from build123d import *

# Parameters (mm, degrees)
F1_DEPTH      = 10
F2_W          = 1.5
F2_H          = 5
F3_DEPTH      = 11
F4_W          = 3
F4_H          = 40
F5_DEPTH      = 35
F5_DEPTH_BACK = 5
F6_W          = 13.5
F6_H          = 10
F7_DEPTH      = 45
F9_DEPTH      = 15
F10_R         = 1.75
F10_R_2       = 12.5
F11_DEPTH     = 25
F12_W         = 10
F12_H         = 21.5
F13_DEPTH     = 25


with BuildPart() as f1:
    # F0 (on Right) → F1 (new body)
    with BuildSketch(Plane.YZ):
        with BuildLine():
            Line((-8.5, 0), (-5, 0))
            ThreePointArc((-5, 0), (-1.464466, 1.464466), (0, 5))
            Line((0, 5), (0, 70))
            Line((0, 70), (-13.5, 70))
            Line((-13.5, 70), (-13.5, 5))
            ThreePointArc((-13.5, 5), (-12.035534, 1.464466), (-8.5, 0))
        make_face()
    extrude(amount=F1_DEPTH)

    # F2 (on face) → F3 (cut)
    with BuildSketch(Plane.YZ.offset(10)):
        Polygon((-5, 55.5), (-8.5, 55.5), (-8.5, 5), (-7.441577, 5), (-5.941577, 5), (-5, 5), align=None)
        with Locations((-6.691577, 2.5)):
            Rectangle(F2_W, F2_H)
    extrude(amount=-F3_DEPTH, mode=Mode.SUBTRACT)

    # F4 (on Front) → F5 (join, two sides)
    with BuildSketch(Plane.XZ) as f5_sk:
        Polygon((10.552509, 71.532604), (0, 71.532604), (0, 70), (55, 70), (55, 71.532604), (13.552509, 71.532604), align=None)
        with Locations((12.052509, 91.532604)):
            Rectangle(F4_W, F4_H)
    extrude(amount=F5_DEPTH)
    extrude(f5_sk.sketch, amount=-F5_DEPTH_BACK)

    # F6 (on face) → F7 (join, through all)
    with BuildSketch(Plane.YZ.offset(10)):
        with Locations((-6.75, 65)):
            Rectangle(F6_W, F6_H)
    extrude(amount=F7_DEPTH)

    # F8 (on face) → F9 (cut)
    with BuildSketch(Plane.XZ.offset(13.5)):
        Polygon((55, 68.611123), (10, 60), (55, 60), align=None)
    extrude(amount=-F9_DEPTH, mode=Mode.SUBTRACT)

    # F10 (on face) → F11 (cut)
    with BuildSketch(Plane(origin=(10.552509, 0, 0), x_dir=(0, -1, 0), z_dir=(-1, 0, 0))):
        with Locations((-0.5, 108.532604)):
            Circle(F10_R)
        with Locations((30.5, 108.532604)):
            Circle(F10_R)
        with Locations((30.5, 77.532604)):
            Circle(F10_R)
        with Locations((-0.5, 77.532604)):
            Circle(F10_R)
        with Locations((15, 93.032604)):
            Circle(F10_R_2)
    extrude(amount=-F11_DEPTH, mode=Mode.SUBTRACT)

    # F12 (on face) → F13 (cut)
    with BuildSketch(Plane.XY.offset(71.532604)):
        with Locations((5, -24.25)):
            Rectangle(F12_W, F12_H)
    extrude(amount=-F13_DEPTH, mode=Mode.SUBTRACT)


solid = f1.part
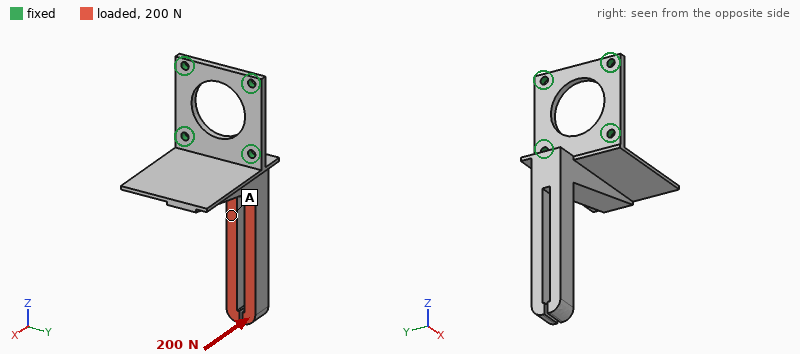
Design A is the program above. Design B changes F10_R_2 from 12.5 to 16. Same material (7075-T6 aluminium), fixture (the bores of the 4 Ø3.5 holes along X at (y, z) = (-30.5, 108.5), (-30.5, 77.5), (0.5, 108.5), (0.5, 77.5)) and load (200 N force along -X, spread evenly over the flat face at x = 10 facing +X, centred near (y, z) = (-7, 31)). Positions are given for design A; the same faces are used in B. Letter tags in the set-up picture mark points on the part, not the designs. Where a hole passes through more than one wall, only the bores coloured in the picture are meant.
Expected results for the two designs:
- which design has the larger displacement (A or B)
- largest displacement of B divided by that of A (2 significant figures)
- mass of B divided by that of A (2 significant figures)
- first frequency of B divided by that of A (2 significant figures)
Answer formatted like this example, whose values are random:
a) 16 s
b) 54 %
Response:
a) B
b) 1.1
c) 0.95
d) 0.95
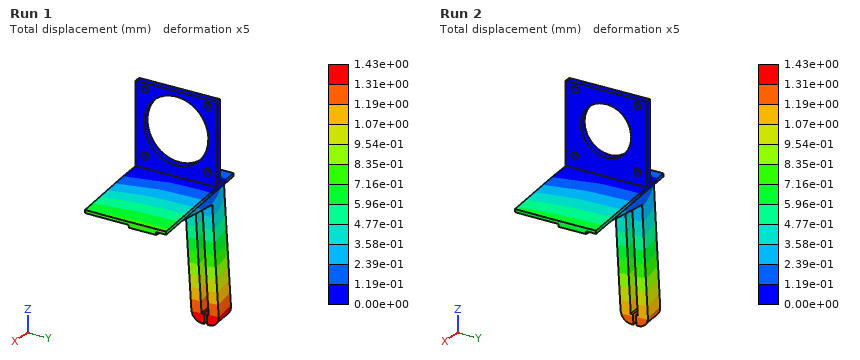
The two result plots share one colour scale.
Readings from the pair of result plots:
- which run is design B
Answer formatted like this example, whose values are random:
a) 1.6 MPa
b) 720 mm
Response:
a) Run 1
